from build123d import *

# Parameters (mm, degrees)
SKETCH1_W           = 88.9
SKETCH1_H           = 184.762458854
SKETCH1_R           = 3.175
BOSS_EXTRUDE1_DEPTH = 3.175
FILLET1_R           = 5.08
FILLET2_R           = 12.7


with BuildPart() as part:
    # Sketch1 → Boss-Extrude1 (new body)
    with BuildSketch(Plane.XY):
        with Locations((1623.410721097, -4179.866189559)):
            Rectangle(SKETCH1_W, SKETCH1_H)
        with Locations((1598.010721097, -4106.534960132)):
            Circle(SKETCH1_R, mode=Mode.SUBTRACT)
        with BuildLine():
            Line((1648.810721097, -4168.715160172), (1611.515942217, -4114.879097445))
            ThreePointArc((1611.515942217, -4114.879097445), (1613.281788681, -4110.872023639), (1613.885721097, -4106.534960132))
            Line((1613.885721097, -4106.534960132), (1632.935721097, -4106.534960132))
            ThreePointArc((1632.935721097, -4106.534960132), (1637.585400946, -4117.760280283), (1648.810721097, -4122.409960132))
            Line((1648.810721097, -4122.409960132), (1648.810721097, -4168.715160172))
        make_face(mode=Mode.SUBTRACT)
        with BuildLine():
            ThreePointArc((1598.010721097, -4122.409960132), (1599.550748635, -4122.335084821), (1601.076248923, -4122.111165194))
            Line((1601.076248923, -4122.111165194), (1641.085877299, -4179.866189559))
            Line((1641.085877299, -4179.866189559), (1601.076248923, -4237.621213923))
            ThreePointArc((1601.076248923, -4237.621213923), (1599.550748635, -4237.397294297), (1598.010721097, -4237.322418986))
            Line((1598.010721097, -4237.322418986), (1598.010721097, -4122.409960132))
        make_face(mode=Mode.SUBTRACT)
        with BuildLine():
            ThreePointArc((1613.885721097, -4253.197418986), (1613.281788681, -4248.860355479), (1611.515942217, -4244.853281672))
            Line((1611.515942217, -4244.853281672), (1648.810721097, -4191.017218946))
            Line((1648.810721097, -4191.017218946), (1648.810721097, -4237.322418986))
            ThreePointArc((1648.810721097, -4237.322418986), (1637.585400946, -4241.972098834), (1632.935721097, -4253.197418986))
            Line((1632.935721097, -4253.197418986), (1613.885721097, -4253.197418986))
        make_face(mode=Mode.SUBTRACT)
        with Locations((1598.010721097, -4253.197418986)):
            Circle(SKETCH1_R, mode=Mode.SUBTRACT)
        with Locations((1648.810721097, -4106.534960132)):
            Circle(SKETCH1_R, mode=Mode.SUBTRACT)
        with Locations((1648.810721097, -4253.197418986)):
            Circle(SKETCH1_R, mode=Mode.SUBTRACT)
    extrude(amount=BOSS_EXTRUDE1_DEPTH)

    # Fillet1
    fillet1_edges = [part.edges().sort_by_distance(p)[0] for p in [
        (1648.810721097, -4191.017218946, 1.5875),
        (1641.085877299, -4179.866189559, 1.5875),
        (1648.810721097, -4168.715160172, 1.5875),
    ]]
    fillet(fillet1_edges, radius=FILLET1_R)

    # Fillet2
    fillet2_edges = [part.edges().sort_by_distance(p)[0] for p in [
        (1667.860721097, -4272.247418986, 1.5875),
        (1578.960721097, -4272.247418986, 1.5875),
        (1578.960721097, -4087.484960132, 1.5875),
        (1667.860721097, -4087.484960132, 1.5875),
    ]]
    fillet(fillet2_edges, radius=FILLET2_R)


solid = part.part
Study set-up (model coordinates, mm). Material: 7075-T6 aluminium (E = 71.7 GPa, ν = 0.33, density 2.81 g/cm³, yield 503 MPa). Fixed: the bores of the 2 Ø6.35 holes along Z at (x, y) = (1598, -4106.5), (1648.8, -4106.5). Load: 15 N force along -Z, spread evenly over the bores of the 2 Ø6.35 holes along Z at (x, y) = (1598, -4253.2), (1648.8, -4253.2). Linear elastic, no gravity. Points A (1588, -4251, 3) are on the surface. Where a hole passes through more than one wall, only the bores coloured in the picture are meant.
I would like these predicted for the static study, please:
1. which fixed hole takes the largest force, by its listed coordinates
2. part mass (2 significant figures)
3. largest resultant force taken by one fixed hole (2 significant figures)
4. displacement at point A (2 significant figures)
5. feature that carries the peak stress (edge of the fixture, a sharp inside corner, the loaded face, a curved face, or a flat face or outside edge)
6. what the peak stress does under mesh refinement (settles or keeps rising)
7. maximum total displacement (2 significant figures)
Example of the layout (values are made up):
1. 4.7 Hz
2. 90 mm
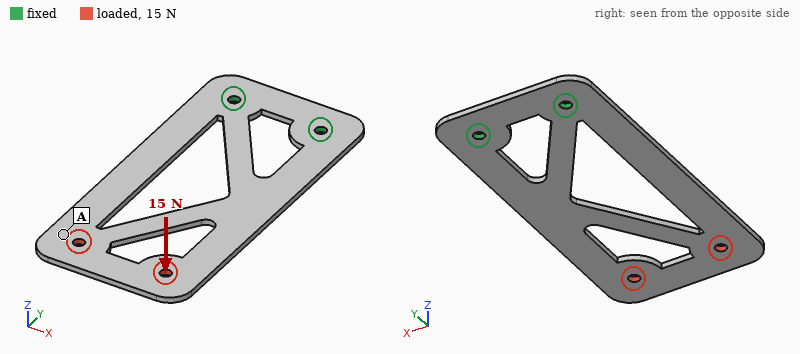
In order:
1. (1598, -4106.5)
2. 100 g
3. 9.1 N
4. 1.5 mm
5. edge of the fixture
6. keeps rising
7. 1.9 mm
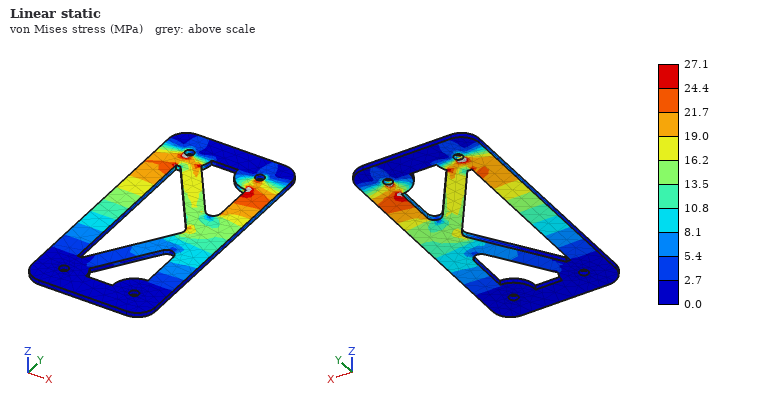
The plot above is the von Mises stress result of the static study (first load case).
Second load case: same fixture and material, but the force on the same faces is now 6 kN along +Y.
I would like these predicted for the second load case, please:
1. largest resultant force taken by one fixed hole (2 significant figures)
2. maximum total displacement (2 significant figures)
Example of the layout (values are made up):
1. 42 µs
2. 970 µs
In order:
1. 3.2 kN
2. 0.15 mm
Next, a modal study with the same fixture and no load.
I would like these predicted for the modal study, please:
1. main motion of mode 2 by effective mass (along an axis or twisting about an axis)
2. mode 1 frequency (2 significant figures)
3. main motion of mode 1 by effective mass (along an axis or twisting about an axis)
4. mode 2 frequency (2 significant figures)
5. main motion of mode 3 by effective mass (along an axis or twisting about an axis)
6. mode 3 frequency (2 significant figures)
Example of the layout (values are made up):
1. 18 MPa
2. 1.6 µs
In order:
1. twisting about Y
2. 83 Hz
3. along Z
4. 300 Hz
5. along Z
6. 550 Hz
